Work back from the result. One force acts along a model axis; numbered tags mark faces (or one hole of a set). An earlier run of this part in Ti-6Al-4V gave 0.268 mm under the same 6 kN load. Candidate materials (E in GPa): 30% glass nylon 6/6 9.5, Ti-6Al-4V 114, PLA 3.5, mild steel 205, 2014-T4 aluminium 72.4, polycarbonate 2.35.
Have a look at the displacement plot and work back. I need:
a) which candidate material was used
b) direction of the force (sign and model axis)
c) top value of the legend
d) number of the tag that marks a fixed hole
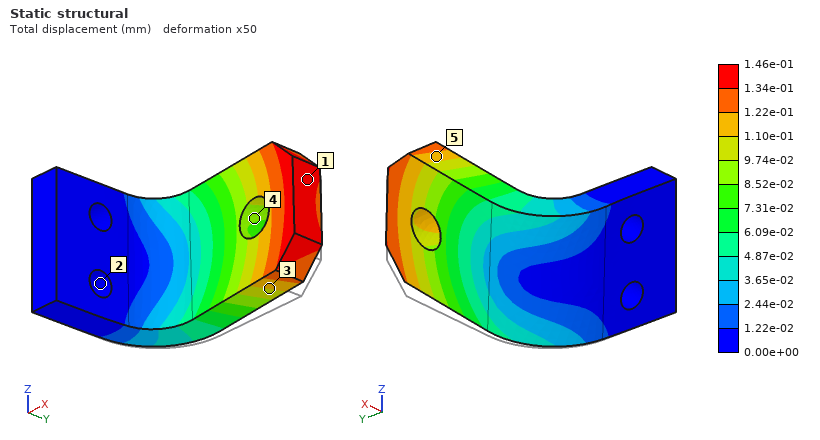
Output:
mild steel
+Z
1.46e-01 mm
2
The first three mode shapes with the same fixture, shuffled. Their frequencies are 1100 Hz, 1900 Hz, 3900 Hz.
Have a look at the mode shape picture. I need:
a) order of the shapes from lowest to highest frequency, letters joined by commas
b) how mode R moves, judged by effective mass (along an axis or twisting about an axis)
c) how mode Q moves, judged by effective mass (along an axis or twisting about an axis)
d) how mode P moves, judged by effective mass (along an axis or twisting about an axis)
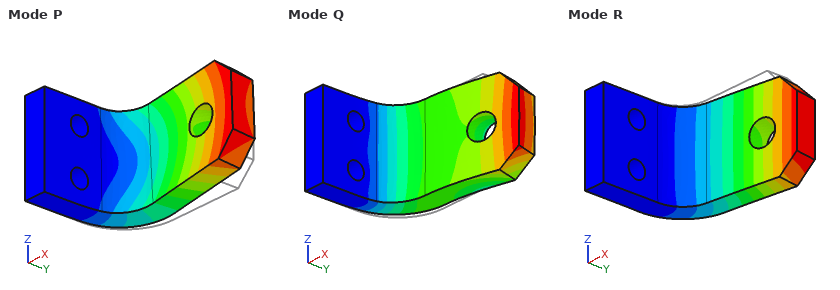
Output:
R, P, Q
along Y
along X
along Z
